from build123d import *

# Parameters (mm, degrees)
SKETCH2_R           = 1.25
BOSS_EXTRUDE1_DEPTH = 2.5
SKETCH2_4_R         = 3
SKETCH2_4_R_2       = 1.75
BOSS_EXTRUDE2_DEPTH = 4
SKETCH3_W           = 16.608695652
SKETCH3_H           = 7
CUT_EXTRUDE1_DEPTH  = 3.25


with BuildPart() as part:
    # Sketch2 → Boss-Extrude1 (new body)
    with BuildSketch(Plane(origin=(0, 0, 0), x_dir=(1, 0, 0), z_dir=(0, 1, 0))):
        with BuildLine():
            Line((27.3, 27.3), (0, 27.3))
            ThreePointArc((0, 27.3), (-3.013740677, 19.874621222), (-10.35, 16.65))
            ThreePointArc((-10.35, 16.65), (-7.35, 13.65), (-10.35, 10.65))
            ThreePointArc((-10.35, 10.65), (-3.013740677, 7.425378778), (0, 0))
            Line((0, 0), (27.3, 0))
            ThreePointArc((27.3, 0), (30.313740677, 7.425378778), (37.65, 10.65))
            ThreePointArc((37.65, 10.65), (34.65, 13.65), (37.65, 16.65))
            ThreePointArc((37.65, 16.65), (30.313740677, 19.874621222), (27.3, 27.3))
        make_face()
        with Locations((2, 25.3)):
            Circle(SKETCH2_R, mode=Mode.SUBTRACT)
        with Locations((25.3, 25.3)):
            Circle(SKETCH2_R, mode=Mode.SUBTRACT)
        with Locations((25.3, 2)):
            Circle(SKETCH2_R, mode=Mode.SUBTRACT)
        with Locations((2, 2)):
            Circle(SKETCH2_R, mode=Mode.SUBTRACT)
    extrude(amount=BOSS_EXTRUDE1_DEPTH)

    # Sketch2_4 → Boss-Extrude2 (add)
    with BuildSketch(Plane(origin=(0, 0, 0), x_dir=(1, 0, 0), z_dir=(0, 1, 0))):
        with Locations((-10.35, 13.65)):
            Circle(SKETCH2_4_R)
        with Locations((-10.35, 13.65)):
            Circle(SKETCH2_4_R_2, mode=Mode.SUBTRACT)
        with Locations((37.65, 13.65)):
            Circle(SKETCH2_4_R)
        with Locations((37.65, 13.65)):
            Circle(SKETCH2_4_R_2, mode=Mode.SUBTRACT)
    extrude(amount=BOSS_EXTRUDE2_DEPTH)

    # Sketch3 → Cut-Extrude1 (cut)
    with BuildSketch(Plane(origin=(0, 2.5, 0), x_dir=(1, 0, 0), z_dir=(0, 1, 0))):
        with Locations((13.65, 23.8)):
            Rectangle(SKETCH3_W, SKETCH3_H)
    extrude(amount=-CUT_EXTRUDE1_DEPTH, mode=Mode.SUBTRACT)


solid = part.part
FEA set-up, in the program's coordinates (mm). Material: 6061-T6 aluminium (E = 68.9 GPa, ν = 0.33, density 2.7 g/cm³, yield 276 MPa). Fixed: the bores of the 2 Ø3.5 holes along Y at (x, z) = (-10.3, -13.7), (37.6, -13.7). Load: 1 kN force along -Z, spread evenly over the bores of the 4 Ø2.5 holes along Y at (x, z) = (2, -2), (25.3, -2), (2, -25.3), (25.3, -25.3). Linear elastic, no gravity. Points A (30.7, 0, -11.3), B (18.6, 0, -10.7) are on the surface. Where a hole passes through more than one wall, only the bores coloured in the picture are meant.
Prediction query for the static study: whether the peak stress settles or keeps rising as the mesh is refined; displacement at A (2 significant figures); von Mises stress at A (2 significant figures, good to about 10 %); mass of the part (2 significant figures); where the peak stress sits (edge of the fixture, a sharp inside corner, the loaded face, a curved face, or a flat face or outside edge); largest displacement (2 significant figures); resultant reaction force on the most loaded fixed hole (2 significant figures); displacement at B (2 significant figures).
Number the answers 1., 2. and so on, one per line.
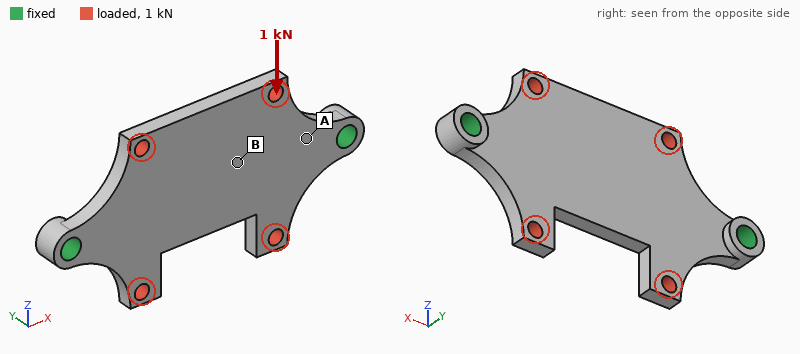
1. keeps rising
2. 11 µm
3. 32 MPa
4. 5.8 g
5. edge of the fixture
6. 21 µm
7. 510 N
8. 19 µm
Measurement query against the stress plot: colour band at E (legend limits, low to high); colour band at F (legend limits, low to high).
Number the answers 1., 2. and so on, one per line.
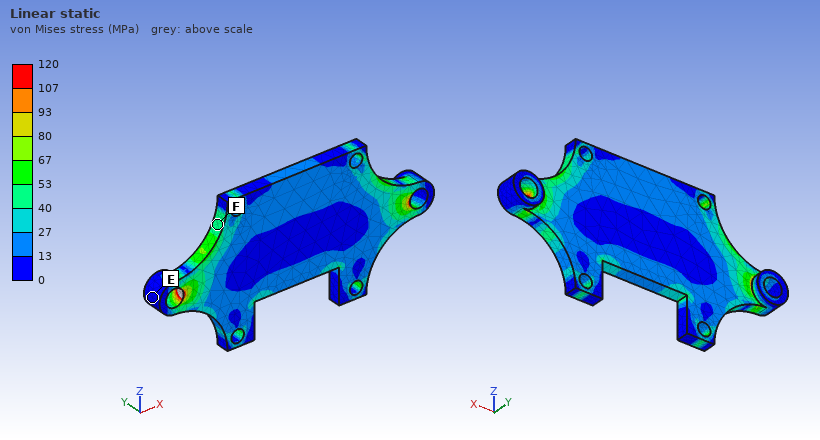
1. 0 to 13 MPa
2. 40 to 53 MPa
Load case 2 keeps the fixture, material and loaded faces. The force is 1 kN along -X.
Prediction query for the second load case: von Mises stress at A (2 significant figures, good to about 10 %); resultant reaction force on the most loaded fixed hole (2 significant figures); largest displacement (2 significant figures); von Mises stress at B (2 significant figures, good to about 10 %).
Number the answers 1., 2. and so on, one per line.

1. 18 MPa
2. 500 N
3. 21 µm
4. 9.0 MPa
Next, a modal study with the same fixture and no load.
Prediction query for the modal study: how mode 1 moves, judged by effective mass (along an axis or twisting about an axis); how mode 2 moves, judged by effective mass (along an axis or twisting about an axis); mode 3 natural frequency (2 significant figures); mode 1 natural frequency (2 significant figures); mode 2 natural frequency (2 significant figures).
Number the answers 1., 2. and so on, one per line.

1. along Y
2. along Y
3. 11 kHz
4. 4300 Hz
5. 5700 Hz
